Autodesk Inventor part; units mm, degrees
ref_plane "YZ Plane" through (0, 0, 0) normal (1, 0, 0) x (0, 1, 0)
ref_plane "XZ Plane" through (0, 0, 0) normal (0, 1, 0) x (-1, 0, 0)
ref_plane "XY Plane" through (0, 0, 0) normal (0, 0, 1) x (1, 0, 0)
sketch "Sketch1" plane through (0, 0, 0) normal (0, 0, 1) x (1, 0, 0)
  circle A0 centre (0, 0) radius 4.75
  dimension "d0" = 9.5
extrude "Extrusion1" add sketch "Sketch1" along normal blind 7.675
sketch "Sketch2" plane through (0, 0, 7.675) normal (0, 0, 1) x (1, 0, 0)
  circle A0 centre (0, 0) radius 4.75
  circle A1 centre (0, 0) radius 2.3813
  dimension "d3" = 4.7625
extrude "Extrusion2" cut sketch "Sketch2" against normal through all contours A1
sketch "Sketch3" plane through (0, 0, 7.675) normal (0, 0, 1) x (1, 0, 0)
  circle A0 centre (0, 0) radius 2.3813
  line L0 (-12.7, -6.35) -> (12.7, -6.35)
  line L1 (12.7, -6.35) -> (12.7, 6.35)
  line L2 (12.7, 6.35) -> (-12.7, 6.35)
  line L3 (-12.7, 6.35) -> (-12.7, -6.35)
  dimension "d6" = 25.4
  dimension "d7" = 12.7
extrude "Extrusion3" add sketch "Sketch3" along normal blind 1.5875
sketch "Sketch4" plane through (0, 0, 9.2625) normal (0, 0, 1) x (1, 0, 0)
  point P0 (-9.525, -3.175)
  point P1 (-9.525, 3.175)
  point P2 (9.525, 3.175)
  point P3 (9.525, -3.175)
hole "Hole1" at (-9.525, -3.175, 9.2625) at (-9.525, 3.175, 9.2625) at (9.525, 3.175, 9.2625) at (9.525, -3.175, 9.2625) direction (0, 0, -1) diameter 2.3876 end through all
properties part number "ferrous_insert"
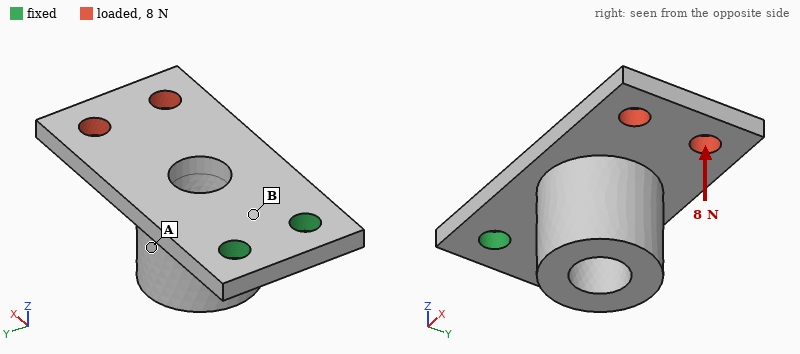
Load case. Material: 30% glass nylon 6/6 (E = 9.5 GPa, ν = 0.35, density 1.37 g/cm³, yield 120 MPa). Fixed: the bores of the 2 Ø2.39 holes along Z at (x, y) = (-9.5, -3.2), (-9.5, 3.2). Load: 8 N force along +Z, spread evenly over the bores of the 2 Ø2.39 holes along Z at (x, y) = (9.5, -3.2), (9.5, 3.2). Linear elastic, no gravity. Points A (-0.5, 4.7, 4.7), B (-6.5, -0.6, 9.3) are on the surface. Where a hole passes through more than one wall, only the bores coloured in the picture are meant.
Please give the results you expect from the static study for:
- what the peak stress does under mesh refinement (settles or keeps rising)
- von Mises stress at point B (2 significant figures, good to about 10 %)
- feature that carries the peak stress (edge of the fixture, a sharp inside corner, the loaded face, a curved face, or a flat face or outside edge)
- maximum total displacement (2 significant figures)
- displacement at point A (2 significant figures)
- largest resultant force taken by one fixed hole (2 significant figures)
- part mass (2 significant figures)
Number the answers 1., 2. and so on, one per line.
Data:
1. keeps rising
2. 21 MPa
3. edge of the fixture
4. 0.34 mm
5. 0.11 mm
6. 4.8 N
7. 1.2 g
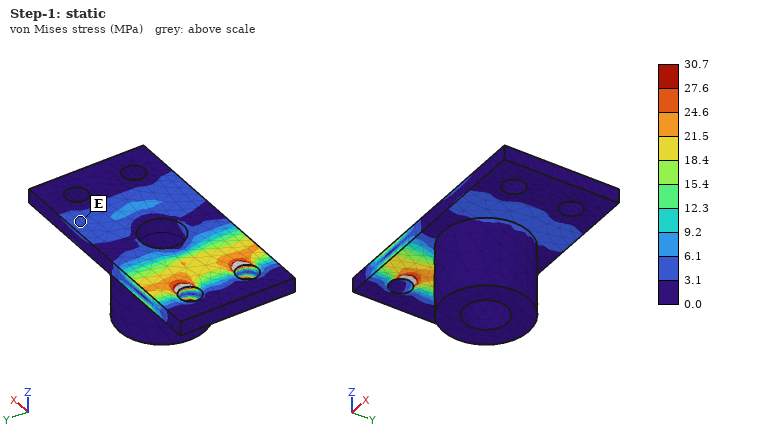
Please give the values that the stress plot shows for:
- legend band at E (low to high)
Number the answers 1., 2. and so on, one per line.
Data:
1. 3.1 to 6.1 MPa
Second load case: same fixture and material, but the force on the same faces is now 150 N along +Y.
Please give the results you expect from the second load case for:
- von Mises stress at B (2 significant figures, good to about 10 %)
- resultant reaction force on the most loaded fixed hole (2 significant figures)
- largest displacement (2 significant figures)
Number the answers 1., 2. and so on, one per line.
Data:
1. 30 MPa
2. 360 N
3. 0.26 mm
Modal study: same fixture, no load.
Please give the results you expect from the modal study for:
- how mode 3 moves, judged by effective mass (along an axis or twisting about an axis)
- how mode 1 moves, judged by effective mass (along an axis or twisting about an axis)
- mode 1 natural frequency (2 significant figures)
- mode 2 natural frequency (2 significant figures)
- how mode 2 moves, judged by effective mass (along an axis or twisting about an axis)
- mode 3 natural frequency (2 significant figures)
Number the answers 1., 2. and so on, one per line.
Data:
1. along Y
2. along Z
3. 1400 Hz
4. 4800 Hz
5. along Y
6. 7700 Hz
